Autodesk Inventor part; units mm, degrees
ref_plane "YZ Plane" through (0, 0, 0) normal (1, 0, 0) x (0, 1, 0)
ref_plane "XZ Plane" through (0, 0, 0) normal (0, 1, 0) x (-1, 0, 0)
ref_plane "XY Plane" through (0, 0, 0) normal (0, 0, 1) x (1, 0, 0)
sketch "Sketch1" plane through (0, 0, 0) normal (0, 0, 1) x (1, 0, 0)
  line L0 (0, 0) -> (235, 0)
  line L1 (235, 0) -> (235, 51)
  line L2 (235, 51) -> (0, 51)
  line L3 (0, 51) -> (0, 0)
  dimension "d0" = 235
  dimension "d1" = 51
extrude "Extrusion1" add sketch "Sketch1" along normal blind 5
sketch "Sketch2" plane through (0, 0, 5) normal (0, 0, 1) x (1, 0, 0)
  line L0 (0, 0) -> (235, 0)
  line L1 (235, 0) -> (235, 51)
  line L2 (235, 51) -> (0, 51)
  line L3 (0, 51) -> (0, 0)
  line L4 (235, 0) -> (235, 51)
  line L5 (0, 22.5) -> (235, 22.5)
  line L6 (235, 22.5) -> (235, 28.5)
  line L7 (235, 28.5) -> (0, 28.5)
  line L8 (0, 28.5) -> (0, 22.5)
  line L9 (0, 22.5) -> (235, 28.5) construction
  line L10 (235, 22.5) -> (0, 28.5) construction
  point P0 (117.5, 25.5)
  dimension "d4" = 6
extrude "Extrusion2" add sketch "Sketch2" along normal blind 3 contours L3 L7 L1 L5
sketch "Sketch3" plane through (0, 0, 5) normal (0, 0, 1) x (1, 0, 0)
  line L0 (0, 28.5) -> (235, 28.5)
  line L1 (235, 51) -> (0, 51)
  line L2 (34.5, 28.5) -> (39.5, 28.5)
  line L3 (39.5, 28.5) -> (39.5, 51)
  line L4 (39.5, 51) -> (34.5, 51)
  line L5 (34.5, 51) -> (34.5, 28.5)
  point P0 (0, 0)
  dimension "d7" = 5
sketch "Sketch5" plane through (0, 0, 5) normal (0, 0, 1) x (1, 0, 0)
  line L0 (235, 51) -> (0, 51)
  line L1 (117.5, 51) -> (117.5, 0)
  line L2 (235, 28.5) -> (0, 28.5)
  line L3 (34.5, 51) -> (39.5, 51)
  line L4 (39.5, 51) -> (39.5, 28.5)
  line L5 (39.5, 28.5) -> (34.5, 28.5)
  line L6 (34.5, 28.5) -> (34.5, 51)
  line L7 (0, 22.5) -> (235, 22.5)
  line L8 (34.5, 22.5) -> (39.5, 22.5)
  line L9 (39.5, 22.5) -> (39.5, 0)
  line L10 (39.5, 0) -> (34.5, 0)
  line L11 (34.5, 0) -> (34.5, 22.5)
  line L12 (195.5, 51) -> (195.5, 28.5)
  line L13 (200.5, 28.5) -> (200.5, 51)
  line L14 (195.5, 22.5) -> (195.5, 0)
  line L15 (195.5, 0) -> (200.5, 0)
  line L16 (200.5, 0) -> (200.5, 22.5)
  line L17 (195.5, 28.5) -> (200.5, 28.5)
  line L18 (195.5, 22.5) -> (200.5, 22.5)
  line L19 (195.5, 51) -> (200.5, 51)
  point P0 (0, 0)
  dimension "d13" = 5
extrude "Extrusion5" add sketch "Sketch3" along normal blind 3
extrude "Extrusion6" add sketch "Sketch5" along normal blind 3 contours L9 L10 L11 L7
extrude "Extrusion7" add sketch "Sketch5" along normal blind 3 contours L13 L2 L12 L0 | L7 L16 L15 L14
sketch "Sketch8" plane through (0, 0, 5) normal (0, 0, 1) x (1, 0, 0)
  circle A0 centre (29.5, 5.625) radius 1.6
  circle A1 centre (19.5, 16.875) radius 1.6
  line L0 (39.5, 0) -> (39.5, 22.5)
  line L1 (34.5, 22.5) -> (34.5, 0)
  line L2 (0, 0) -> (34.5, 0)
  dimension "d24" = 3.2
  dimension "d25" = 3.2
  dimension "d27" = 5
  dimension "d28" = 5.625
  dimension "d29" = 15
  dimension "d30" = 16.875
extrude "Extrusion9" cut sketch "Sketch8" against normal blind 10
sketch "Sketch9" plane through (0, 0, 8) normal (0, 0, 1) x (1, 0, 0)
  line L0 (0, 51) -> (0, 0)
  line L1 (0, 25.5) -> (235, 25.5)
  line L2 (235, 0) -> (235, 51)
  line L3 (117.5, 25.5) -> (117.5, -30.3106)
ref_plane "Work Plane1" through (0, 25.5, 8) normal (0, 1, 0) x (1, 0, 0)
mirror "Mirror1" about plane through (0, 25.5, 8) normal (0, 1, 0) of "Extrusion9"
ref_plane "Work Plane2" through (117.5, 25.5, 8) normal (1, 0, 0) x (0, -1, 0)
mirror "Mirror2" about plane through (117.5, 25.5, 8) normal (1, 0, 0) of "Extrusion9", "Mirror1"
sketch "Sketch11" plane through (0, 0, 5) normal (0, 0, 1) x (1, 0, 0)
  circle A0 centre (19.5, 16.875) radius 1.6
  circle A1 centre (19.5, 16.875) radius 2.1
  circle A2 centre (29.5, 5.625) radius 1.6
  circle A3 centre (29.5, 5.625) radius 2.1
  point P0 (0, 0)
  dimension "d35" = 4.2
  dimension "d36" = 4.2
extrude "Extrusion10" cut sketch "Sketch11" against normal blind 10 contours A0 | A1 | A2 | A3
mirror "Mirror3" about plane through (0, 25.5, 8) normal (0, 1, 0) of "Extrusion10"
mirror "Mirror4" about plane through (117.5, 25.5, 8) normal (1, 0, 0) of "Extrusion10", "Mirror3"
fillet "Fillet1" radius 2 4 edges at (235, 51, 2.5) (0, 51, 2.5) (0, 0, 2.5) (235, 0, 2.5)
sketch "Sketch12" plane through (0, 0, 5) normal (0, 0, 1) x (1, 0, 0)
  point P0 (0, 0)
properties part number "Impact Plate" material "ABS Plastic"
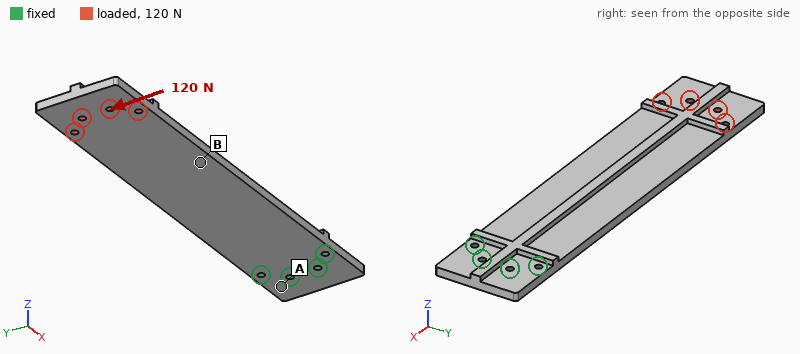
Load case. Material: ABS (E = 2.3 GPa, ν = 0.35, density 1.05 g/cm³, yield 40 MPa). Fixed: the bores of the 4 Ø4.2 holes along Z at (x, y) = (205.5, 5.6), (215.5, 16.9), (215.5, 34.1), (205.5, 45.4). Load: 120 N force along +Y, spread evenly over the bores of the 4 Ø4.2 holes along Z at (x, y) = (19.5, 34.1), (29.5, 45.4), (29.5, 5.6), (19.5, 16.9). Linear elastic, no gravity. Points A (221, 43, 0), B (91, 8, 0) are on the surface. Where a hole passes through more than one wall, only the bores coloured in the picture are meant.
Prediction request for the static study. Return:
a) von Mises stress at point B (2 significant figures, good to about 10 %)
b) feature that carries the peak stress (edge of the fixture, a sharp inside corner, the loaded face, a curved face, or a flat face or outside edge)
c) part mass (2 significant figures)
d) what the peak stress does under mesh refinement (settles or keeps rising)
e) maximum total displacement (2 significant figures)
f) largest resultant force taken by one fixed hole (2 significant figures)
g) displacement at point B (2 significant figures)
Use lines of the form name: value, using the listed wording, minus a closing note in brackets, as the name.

von Mises stress at point B: 2.6 MPa
feature that carries the peak stress: edge of the fixture
part mass: 68 g
what the peak stress does under mesh refinement: keeps rising
maximum total displacement: 2.4 mm
largest resultant force taken by one fixed hole: 490 N
displacement at point B: 0.99 mm
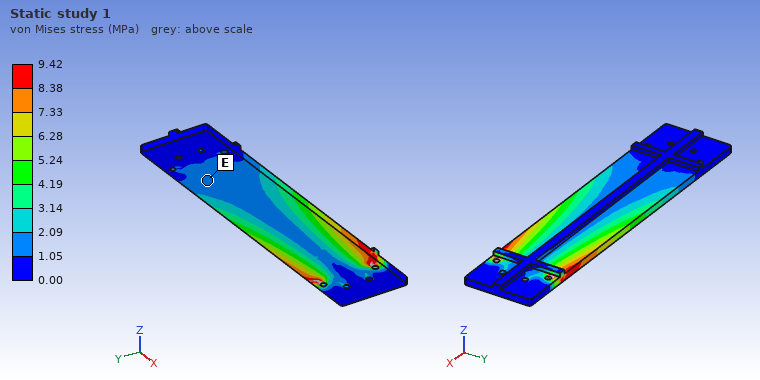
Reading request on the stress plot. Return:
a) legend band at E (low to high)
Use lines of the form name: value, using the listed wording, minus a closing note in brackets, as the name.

legend band at E: 1.05 to 2.09 MPa
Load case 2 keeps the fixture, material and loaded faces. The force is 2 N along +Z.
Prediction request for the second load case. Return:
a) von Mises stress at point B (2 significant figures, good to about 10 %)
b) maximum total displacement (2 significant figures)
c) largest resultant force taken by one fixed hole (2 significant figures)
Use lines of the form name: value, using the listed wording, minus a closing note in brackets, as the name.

von Mises stress at point B: 0.46 MPa
maximum total displacement: 2.6 mm
largest resultant force taken by one fixed hole: 8.2 N
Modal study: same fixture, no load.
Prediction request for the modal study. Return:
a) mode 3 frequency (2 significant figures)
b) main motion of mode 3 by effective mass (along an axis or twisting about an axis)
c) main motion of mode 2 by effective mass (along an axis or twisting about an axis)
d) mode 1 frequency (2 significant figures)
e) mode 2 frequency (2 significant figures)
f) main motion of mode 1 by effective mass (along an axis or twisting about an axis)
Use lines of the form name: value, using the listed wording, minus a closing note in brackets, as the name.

mode 3 frequency: 240 Hz
main motion of mode 3 by effective mass: twisting about X
main motion of mode 2 by effective mass: along Z
mode 1 frequency: 33 Hz
mode 2 frequency: 210 Hz
main motion of mode 1 by effective mass: along Z
